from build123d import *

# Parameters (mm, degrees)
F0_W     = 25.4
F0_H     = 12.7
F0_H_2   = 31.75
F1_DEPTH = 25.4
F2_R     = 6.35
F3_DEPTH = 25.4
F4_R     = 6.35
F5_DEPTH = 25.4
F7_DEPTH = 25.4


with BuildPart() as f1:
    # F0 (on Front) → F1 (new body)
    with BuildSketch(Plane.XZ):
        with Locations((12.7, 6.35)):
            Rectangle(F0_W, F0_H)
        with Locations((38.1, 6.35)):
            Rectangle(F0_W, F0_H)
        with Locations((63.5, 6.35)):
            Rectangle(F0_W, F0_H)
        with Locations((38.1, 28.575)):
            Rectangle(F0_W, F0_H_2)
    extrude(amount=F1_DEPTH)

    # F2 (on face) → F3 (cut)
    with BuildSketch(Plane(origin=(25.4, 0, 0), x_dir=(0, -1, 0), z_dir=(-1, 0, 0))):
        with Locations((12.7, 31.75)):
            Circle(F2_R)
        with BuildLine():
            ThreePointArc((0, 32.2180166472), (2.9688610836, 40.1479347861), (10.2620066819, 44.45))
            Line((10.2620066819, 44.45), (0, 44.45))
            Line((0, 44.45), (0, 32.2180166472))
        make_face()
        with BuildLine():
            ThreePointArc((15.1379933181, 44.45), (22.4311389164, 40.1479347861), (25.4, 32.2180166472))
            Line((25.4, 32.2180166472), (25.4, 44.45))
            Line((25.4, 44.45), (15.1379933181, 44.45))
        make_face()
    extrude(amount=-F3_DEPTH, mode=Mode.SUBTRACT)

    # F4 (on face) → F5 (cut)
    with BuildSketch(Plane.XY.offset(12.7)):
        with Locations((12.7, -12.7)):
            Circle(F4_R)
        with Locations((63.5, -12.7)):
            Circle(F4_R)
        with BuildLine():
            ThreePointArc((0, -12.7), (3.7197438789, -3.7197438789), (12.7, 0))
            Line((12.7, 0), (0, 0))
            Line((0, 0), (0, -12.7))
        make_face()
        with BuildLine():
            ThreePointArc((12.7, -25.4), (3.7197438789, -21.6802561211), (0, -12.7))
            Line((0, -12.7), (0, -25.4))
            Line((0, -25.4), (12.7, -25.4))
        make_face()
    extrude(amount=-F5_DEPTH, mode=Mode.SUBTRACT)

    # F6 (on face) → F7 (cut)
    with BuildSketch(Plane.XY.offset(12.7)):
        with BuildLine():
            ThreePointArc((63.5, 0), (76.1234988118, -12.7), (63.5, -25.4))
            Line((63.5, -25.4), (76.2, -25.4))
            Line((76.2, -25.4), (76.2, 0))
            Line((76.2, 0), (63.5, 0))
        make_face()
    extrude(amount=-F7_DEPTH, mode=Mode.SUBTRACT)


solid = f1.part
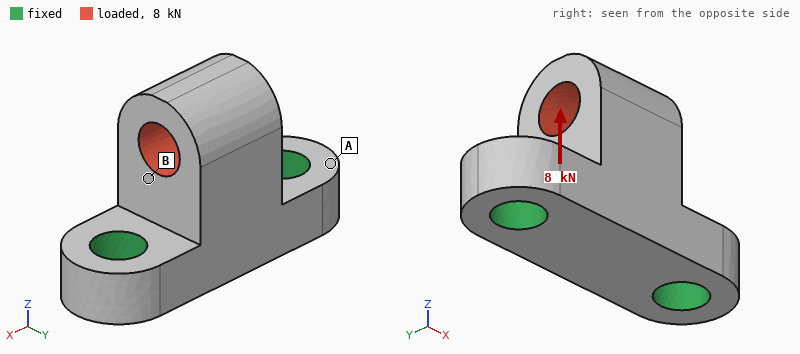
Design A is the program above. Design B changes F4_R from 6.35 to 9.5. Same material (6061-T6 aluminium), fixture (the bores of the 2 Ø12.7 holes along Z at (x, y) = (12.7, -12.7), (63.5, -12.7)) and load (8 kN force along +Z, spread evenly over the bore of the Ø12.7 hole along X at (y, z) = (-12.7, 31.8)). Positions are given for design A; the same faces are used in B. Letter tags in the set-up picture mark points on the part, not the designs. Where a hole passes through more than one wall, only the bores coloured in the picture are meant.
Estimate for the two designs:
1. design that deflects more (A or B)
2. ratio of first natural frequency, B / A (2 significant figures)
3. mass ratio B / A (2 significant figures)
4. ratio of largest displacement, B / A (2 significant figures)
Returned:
A
1.2
0.89
0.79
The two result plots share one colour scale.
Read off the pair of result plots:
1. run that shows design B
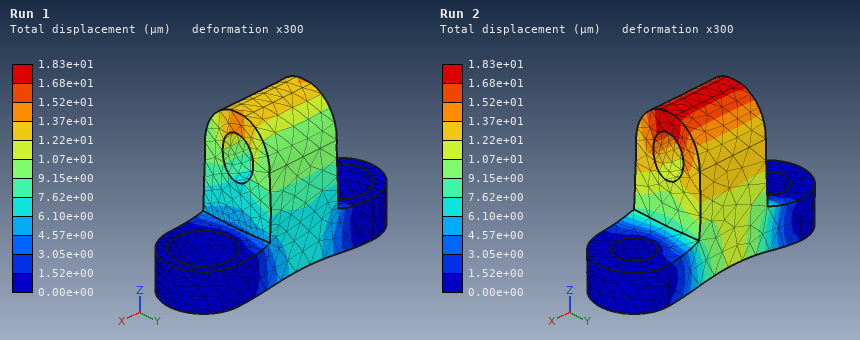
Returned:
Run 1
